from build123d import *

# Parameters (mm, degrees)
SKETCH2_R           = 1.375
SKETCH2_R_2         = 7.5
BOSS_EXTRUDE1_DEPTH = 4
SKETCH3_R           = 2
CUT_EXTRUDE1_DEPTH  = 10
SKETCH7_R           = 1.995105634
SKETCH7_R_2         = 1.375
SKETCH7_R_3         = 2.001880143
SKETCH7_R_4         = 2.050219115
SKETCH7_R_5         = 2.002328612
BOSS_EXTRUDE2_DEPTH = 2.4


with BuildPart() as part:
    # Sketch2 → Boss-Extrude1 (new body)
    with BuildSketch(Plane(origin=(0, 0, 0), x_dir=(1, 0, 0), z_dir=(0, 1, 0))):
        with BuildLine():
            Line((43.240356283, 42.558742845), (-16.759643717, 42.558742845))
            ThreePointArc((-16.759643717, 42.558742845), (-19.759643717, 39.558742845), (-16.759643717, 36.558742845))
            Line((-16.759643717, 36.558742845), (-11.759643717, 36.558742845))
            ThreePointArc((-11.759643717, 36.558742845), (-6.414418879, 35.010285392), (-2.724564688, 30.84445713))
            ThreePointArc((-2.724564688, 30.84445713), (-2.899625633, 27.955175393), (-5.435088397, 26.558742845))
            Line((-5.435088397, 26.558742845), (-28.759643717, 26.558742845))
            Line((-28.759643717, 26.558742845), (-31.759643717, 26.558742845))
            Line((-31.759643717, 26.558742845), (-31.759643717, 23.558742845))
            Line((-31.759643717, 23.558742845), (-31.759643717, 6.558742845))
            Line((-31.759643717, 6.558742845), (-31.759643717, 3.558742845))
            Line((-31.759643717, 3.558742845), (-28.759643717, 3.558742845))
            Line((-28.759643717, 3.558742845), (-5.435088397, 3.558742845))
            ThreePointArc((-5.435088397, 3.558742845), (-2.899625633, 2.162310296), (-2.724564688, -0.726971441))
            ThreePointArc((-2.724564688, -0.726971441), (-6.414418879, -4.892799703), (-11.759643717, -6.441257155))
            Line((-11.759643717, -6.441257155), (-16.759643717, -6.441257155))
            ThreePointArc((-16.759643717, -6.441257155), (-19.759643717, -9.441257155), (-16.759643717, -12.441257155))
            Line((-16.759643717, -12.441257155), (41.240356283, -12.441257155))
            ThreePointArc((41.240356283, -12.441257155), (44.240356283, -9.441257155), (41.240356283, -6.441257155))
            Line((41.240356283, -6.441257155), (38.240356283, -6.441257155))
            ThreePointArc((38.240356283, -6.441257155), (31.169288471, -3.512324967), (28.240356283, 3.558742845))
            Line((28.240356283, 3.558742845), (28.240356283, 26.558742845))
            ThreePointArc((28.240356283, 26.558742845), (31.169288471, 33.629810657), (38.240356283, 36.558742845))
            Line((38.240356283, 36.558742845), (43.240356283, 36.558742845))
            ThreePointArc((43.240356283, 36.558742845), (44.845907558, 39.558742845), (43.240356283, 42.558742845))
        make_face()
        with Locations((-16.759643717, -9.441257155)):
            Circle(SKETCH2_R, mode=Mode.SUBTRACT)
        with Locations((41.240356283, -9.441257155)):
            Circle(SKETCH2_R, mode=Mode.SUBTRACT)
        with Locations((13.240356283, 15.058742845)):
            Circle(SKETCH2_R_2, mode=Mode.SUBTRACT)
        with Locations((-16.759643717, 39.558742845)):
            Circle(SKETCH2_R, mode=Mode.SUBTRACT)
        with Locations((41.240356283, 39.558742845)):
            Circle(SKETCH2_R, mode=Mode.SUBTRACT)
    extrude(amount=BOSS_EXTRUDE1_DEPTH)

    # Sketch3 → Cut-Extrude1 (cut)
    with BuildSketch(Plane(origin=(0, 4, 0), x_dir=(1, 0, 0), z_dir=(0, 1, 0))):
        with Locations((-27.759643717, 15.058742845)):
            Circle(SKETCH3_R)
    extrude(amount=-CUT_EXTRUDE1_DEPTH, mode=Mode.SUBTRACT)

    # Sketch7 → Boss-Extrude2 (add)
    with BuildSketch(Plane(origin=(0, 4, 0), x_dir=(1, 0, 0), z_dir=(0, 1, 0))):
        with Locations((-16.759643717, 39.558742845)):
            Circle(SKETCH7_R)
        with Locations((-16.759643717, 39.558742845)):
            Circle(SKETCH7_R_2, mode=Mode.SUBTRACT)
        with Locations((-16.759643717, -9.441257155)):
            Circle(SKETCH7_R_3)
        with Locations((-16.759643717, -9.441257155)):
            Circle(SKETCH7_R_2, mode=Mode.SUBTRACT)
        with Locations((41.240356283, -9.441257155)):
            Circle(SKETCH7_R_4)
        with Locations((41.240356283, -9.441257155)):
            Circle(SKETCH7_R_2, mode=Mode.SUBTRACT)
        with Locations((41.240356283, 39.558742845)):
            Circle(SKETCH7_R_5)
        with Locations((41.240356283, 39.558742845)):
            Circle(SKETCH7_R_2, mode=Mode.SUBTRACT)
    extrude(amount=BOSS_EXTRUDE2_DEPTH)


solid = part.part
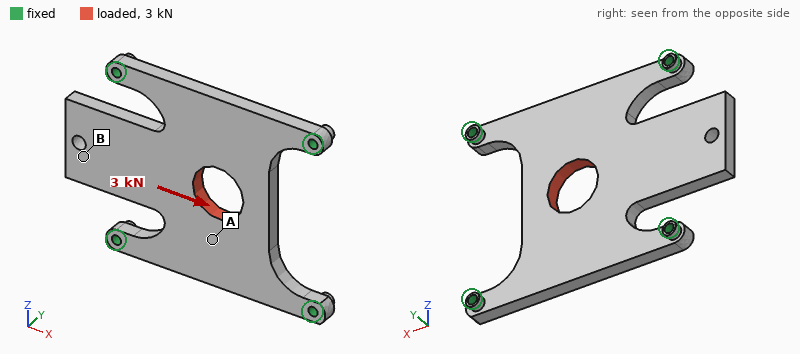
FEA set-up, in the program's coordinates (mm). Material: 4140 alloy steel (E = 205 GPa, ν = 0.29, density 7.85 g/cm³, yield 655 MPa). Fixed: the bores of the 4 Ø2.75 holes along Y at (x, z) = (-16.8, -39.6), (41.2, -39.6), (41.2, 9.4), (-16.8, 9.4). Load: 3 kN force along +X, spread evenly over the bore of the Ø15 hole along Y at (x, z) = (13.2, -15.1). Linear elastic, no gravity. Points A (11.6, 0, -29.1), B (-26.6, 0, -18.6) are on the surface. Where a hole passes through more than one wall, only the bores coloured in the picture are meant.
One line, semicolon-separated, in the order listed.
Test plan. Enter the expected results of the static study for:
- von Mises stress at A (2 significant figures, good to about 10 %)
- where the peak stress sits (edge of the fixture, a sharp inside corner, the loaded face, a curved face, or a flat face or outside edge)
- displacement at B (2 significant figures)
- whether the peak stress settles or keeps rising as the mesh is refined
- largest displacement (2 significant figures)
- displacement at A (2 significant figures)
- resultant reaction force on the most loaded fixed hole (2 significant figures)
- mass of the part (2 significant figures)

24 MPa; edge of the fixture; 4.9 µm; keeps rising; 7.0 µm; 4.1 µm; 830 N; 83 g
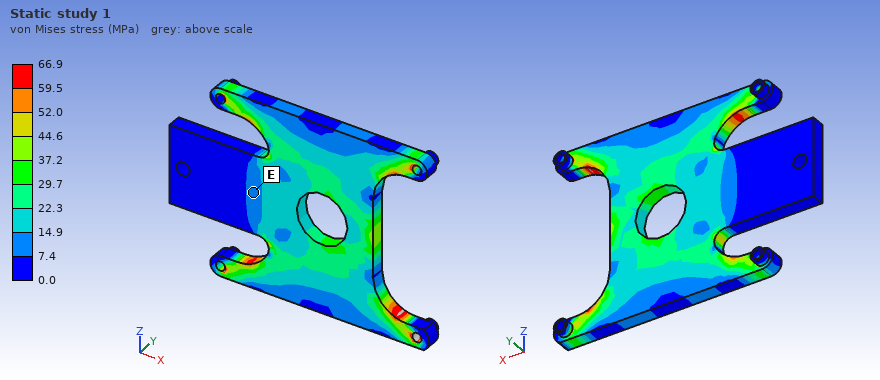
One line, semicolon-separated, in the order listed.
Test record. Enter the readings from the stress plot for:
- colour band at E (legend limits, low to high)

7.4 to 14.9 MPa
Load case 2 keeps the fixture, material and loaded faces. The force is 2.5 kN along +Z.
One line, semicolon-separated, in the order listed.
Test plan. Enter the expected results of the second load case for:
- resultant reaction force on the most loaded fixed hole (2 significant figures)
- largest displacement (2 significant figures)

910 N; 14 µm
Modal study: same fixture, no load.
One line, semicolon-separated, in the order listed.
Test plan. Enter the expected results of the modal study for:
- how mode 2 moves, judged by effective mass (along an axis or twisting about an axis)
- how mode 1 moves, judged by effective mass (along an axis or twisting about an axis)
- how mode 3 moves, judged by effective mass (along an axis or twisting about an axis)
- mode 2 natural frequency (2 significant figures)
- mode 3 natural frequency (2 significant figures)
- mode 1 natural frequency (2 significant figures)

along Y; along Y; twisting about X; 3600 Hz; 5700 Hz; 1900 Hz
